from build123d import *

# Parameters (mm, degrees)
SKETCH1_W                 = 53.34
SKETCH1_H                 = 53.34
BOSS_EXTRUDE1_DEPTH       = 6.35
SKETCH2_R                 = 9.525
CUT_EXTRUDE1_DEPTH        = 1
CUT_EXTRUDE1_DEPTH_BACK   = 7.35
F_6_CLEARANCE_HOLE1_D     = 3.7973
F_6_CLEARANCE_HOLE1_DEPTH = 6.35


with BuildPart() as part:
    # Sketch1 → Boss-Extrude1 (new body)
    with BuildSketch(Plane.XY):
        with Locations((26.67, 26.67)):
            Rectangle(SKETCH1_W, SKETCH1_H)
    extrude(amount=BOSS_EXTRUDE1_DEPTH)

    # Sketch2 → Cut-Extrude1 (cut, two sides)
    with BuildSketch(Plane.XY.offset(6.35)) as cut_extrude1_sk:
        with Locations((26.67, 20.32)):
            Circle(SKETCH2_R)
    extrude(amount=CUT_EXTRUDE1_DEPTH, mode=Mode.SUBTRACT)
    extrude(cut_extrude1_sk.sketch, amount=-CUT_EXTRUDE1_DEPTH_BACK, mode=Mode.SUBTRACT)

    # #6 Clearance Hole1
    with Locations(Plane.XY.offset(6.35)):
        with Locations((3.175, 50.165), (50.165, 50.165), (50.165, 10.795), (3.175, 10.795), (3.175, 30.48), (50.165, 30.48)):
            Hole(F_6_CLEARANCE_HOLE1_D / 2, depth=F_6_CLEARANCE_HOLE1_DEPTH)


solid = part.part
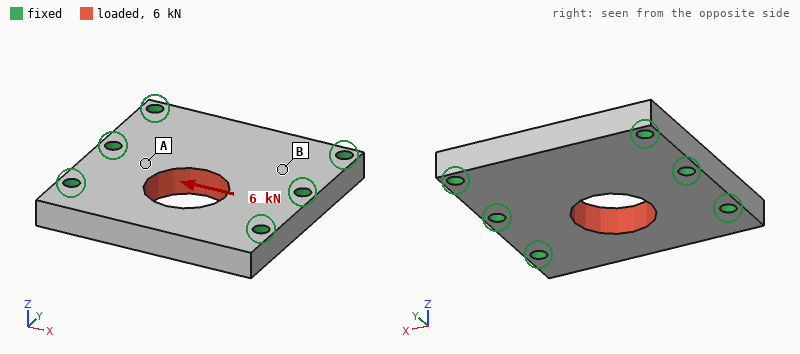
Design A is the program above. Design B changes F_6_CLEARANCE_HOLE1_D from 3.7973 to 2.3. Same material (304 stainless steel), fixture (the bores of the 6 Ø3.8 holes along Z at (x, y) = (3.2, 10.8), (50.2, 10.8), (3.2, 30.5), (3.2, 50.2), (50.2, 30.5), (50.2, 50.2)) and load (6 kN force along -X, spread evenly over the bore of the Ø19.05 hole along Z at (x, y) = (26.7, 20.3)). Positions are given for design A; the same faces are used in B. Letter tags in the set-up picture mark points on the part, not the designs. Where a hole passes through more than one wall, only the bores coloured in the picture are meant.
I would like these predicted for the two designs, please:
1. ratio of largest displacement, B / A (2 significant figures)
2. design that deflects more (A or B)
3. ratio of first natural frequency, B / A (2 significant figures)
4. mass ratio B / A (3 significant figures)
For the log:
1.1
B
0.89
1.02
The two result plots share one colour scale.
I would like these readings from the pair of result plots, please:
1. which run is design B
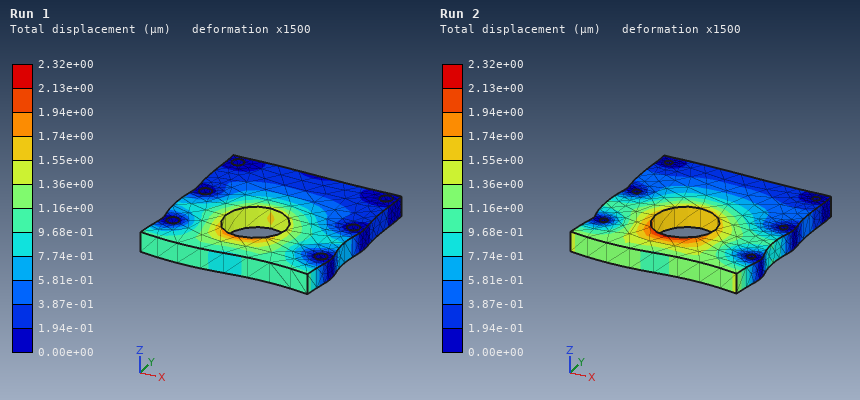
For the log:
Run 2
